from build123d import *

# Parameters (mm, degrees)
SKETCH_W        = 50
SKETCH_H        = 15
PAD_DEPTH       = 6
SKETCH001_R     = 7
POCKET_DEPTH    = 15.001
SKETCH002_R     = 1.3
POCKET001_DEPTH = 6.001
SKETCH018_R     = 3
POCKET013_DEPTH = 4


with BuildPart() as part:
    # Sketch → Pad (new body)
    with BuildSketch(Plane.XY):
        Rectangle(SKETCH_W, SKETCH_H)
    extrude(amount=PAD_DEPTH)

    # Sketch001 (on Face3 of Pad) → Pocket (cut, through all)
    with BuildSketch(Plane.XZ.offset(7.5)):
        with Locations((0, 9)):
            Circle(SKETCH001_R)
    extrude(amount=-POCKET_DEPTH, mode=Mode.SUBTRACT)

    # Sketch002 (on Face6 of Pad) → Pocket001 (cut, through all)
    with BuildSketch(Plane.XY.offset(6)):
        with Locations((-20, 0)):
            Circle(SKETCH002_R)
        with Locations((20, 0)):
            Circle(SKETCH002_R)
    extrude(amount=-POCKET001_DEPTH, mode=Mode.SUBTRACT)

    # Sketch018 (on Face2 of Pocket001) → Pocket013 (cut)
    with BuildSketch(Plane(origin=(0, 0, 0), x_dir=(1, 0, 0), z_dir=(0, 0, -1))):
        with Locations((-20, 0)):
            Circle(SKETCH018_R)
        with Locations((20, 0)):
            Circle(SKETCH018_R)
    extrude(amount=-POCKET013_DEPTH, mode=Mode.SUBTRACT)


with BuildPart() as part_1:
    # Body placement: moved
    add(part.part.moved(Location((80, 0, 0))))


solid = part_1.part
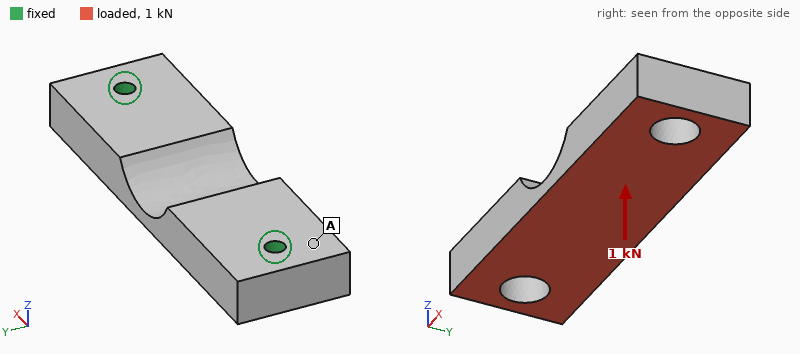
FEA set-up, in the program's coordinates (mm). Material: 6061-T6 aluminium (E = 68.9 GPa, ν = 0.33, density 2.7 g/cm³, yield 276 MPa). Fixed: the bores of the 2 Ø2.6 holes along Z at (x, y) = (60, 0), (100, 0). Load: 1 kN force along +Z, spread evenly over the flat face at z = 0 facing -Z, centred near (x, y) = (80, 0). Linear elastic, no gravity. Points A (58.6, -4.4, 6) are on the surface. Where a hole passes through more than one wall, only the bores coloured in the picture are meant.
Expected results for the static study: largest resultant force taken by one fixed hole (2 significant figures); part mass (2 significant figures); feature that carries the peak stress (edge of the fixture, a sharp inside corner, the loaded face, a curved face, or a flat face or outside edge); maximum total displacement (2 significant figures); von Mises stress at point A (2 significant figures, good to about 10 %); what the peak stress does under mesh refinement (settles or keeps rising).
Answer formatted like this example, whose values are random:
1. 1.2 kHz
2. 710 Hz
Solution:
1. 880 N
2. 10 g
3. edge of the fixture
4. 29 µm
5. 18 MPa
6. keeps rising
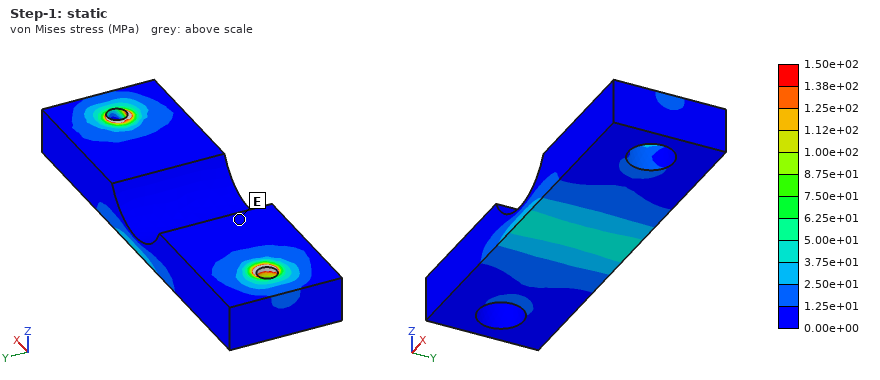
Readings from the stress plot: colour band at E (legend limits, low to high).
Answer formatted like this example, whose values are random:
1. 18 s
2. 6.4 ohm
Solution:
1. 0.00e+00 to 1.25e+01 MPa
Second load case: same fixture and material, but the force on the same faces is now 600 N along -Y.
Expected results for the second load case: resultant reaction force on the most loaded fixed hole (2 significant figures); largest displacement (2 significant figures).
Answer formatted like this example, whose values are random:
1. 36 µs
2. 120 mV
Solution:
1. 300 N
2. 33 µm
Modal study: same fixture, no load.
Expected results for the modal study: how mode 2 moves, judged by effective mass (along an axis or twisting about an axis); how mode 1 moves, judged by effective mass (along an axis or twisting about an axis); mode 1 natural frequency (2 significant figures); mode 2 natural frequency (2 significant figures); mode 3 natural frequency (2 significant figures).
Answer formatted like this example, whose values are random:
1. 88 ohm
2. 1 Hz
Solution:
1. along Z
2. along Y
3. 10 kHz
4. 12 kHz
5. 17 kHz
